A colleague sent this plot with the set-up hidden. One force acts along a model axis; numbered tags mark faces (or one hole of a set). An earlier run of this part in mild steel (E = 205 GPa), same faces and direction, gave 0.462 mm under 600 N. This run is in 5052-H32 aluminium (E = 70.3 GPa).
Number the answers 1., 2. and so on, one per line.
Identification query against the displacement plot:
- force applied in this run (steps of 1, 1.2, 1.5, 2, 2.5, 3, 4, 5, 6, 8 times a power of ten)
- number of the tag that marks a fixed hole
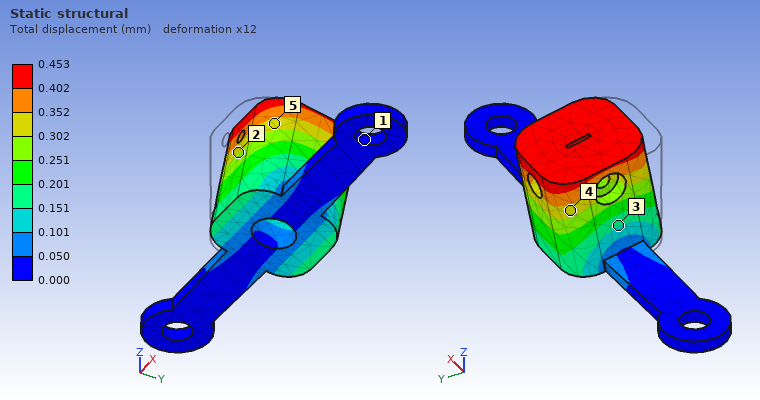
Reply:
1. 200 N
2. 1
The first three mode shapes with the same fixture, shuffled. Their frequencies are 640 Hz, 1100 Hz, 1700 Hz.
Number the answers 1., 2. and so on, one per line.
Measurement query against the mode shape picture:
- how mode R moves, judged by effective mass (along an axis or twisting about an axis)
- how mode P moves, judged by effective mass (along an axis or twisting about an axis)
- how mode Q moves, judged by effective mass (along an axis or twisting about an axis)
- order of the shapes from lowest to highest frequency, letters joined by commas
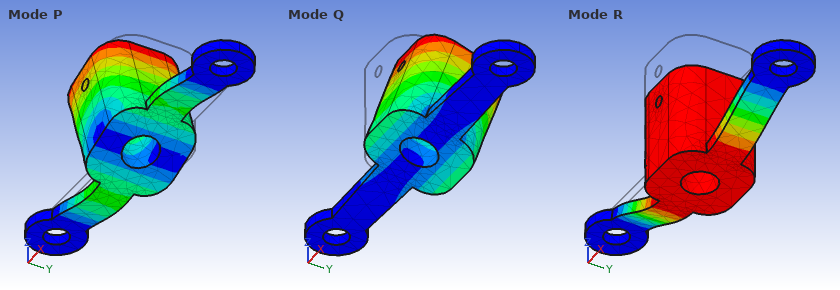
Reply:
1. along Z
2. along X
3. along Y
4. Q, R, P
